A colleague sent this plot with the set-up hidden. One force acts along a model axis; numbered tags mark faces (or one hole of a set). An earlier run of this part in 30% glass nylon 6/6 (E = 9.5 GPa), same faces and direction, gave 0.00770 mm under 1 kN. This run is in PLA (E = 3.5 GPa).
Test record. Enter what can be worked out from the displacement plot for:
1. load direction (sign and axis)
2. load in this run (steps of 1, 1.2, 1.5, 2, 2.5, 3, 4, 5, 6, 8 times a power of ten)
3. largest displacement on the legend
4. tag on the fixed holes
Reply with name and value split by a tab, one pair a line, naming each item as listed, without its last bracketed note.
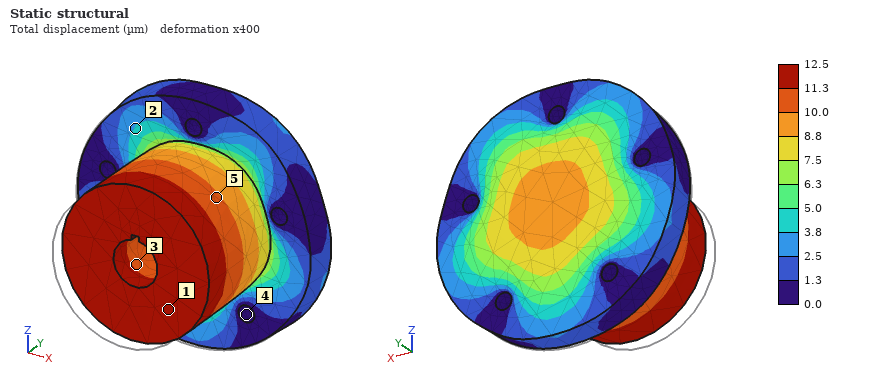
load direction	+Y
load in this run	600 N
largest displacement on the legend	12.5 µm
tag on the fixed holes	4
